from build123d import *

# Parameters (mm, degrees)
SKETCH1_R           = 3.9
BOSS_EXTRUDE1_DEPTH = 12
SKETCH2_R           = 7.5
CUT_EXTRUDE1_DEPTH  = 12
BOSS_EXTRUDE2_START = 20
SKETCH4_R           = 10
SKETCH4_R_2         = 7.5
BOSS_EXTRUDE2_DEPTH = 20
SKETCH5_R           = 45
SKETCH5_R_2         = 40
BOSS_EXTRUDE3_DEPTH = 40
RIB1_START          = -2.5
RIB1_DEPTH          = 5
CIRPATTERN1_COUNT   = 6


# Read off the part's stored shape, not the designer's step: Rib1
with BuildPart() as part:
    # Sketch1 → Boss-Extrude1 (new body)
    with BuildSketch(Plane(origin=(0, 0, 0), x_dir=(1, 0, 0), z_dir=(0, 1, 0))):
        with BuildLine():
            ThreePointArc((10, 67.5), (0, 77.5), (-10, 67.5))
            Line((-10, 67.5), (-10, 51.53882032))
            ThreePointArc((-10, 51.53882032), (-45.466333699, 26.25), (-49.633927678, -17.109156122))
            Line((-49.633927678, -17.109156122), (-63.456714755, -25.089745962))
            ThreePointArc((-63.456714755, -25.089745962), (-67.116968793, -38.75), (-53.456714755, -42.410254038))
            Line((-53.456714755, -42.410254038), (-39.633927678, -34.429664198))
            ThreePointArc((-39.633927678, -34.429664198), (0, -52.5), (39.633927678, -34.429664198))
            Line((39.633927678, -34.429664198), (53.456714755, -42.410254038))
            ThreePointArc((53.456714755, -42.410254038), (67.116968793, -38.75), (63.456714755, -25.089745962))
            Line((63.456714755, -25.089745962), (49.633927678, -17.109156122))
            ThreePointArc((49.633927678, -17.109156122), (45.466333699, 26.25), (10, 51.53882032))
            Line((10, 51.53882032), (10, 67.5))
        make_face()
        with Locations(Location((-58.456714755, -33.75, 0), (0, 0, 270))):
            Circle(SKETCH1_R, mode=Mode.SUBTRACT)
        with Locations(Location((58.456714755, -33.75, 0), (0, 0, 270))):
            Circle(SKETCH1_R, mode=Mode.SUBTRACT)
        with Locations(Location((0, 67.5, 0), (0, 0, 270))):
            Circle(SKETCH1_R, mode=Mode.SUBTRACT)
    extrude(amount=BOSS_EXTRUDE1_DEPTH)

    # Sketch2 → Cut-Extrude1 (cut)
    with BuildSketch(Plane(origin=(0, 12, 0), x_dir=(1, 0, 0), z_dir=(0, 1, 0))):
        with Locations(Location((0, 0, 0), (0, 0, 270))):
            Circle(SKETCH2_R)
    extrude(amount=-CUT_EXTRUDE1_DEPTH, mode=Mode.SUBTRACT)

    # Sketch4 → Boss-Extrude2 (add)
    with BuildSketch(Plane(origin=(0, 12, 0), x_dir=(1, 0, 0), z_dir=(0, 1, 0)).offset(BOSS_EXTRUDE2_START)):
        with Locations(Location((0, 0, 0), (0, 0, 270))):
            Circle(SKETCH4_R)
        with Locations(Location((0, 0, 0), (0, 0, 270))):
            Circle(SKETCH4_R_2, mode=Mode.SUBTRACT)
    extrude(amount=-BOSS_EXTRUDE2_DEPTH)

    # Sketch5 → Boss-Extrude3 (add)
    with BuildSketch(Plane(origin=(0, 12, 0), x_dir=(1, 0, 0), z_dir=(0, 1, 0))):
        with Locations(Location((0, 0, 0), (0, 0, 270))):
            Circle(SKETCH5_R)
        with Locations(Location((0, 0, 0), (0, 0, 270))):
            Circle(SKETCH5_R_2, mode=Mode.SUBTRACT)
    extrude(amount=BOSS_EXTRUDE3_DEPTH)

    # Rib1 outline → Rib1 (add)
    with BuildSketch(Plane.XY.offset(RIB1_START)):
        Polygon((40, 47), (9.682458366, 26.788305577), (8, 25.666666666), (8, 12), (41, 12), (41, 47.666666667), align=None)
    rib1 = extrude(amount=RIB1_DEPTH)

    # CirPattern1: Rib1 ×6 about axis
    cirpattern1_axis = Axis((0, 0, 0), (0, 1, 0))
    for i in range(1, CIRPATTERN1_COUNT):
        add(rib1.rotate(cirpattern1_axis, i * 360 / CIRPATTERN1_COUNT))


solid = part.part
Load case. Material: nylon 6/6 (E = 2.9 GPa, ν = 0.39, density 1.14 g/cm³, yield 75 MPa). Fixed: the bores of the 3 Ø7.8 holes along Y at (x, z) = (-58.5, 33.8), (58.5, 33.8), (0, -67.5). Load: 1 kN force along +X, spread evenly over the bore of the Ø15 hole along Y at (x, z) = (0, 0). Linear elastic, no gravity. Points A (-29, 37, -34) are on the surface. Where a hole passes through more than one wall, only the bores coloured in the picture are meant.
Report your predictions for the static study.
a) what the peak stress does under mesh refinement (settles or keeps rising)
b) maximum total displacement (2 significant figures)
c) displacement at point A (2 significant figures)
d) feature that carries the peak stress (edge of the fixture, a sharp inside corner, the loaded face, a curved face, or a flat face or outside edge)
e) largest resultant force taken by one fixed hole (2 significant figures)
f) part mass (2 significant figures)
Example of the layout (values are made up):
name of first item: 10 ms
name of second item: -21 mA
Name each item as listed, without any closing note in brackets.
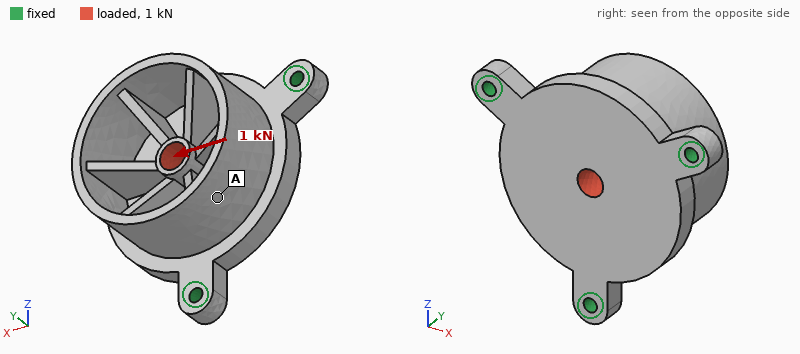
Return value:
what the peak stress does under mesh refinement: keeps rising
maximum total displacement: 90 µm
displacement at point A: 69 µm
feature that carries the peak stress: edge of the fixture
largest resultant force taken by one fixed hole: 470 N
part mass: 220 g
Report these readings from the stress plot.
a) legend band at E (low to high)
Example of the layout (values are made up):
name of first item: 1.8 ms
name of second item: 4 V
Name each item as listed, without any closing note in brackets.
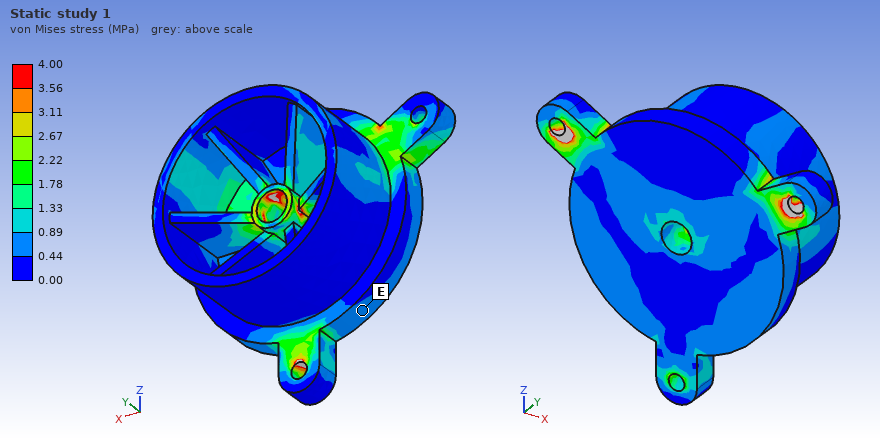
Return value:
legend band at E: 0.44 to 0.89 MPa
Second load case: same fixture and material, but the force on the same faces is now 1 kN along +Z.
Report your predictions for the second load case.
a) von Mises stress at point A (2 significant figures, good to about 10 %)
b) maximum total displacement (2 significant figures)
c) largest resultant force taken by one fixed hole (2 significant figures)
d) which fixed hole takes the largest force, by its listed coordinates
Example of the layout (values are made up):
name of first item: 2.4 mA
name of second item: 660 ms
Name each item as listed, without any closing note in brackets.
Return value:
von Mises stress at point A: 0.54 MPa
maximum total displacement: 100 µm
largest resultant force taken by one fixed hole: 530 N
which fixed hole takes the largest force, by its listed coordinates: (0, -67.5)
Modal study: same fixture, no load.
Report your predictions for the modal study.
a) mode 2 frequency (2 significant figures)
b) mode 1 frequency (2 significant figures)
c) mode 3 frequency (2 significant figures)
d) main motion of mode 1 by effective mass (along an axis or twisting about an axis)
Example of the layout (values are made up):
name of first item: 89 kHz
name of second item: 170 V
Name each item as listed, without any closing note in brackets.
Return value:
mode 2 frequency: 1100 Hz
mode 1 frequency: 1000 Hz
mode 3 frequency: 1100 Hz
main motion of mode 1 by effective mass: along Y
